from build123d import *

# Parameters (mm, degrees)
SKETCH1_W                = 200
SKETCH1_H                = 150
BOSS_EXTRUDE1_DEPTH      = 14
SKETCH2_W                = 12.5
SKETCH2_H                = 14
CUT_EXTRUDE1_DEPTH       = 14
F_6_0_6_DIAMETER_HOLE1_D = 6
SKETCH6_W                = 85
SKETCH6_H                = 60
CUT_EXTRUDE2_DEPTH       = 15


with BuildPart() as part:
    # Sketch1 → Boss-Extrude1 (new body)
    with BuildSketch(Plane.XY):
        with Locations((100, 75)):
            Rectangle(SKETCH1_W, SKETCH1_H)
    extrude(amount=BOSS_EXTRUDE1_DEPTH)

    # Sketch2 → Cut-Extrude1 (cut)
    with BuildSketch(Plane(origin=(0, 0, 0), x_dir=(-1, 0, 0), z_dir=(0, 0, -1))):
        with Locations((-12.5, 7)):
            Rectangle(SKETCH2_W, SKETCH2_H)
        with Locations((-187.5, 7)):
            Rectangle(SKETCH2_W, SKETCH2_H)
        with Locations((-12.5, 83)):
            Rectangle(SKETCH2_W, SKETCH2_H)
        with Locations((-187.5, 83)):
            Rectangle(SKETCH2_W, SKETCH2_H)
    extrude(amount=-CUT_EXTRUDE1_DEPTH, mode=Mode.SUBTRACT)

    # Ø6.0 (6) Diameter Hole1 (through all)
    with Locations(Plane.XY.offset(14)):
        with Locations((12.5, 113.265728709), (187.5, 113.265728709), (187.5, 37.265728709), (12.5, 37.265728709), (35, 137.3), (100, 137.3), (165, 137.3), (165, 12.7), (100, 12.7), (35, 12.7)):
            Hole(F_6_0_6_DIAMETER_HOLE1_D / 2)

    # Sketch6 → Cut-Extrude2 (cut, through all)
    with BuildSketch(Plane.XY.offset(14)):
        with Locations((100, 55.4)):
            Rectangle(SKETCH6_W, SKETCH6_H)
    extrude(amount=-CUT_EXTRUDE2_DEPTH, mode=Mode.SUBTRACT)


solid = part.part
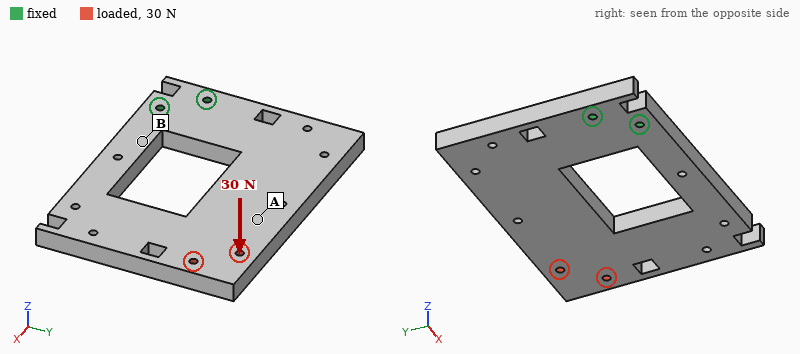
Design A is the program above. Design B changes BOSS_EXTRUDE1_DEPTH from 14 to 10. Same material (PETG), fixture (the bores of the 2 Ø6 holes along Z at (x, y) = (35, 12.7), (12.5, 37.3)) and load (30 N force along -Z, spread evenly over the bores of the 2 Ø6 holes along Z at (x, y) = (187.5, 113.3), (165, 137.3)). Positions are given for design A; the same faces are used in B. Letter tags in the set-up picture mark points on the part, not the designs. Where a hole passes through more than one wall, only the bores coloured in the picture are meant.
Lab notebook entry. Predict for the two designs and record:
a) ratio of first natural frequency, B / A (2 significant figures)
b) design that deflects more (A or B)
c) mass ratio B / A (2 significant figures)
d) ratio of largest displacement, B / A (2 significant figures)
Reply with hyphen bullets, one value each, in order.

- 0.73
- B
- 0.71
- 2.6
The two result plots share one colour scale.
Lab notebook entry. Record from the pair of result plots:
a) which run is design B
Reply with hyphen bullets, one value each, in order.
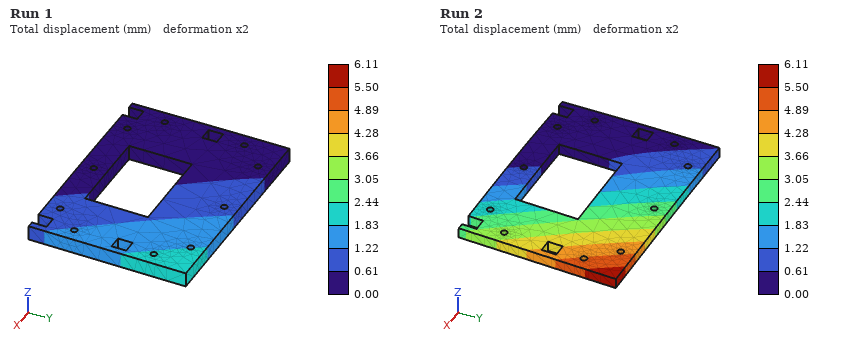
- Run 2
